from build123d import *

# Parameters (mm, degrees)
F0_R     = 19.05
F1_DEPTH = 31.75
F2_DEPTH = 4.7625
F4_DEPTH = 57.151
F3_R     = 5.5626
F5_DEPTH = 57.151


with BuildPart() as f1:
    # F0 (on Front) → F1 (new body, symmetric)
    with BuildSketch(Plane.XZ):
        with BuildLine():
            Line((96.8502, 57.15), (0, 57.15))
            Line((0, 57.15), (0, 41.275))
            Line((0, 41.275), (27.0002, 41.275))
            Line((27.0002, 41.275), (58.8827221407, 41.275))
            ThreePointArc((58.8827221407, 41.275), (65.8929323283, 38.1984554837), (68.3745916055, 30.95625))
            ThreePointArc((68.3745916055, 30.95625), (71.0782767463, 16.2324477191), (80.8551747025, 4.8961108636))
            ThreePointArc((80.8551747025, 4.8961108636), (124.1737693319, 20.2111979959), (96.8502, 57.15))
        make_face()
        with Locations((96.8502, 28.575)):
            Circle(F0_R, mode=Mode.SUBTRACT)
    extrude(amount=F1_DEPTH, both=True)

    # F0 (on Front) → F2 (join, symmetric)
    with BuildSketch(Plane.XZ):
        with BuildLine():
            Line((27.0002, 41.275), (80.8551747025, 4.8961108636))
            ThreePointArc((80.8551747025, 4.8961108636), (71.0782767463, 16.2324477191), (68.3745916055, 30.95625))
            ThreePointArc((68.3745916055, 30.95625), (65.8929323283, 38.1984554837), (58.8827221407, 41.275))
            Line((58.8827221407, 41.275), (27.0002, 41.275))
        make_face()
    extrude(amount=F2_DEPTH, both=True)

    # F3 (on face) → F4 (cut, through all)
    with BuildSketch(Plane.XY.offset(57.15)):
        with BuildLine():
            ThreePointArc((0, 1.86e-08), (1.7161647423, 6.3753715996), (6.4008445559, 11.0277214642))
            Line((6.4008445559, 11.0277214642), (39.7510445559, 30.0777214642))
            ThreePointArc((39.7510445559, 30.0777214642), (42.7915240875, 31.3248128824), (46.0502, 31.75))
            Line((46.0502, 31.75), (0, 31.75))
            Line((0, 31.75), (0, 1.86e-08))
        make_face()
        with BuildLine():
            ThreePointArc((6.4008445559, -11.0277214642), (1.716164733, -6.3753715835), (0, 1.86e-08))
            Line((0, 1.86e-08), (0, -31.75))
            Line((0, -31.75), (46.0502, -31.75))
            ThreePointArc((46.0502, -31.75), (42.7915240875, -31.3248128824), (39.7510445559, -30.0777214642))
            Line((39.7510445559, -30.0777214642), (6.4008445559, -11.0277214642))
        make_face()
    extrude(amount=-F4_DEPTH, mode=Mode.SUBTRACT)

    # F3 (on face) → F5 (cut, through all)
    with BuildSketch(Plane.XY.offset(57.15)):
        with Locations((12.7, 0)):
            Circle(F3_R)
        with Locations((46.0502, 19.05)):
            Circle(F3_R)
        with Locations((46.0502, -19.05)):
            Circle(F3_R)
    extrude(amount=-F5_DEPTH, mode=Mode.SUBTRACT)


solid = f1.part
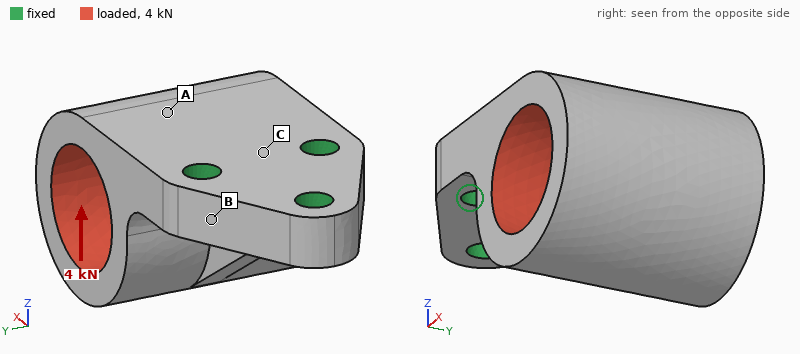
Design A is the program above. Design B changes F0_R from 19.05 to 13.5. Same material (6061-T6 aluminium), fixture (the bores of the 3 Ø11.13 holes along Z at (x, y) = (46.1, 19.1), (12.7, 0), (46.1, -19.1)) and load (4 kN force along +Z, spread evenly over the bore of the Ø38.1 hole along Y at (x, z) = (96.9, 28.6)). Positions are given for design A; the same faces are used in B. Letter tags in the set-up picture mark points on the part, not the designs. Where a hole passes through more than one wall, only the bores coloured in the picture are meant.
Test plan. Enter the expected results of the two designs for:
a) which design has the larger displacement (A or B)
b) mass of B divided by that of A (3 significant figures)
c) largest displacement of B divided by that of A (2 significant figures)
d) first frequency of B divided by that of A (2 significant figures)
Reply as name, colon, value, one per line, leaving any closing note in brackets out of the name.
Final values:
which design has the larger displacement: A
mass of B divided by that of A: 1.23
largest displacement of B divided by that of A: 0.86
first frequency of B divided by that of A: 0.92
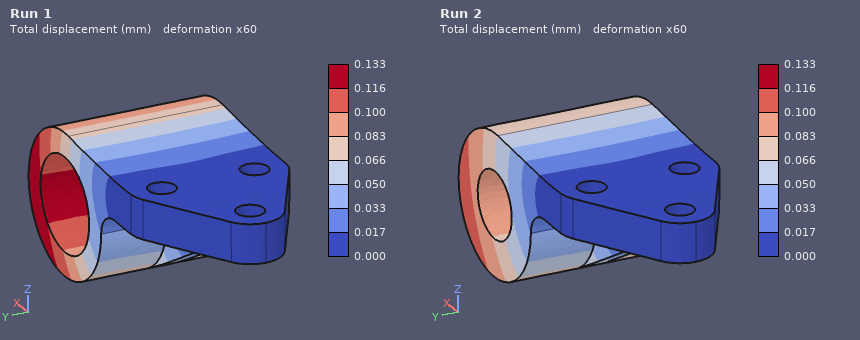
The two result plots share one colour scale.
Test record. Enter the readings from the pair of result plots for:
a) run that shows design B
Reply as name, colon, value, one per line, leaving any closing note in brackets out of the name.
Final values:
run that shows design B: Run 2
